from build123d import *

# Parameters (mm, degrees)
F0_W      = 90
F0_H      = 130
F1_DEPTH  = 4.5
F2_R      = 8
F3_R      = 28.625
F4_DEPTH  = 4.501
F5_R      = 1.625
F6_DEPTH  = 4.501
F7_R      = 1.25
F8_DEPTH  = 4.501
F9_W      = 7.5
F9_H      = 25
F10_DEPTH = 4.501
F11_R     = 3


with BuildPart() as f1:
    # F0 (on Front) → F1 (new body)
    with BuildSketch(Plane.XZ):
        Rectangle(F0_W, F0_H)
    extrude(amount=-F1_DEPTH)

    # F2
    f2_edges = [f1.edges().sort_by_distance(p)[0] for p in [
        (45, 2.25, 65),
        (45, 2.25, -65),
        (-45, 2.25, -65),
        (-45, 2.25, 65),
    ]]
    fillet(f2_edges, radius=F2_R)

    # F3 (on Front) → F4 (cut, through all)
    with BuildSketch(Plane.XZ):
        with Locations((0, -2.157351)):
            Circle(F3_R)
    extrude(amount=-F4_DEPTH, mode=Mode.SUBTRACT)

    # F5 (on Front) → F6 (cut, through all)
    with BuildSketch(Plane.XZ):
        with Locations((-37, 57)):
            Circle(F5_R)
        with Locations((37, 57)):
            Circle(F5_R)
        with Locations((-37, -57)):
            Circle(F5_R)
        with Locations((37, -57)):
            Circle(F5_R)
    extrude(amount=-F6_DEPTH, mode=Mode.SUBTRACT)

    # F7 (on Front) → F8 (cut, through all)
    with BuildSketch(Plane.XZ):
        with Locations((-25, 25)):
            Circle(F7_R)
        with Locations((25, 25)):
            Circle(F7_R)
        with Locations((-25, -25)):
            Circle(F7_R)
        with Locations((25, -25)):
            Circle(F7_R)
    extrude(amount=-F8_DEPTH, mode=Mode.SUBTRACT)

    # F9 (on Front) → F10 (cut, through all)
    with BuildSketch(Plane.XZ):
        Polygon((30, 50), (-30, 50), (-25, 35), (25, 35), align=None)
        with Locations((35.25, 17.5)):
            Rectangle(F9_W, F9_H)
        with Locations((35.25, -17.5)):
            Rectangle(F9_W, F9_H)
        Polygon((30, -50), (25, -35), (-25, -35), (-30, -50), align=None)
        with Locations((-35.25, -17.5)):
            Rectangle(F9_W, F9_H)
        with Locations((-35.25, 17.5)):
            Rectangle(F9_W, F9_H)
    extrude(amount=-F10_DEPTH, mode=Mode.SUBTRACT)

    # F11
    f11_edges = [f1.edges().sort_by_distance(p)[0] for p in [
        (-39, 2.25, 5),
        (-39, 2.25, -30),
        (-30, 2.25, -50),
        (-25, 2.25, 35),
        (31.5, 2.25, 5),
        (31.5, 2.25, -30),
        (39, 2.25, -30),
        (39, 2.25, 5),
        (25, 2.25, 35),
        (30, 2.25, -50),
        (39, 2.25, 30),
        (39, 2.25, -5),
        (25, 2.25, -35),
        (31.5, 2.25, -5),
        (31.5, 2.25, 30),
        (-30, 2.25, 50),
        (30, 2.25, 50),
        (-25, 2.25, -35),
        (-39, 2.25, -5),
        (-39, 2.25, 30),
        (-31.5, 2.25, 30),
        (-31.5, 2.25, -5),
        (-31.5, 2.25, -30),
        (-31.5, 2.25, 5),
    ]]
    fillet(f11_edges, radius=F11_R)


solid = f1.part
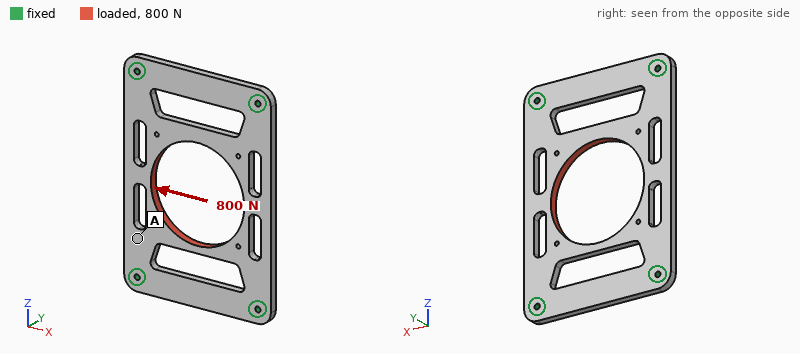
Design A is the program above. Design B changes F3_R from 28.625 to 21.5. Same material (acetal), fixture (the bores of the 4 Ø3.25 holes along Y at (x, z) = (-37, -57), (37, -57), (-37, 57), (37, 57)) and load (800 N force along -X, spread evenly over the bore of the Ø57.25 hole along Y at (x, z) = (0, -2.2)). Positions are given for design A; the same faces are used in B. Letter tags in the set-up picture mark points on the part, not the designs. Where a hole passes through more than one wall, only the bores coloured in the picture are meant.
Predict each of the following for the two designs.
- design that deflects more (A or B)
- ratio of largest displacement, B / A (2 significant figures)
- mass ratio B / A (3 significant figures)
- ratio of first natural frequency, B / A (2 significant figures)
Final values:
A
0.48
1.17
0.88
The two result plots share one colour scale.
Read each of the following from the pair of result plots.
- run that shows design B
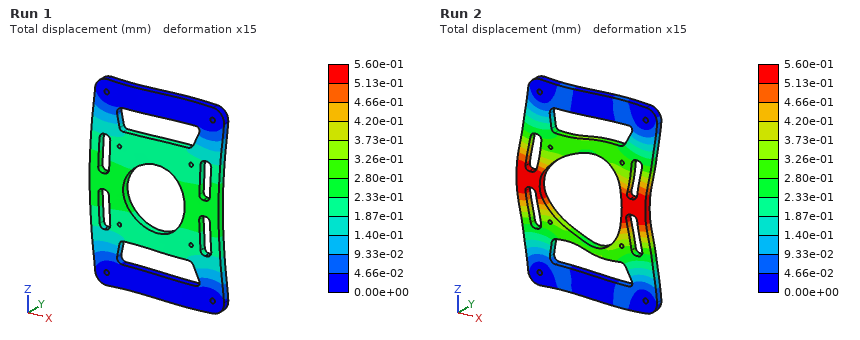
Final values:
Run 1
